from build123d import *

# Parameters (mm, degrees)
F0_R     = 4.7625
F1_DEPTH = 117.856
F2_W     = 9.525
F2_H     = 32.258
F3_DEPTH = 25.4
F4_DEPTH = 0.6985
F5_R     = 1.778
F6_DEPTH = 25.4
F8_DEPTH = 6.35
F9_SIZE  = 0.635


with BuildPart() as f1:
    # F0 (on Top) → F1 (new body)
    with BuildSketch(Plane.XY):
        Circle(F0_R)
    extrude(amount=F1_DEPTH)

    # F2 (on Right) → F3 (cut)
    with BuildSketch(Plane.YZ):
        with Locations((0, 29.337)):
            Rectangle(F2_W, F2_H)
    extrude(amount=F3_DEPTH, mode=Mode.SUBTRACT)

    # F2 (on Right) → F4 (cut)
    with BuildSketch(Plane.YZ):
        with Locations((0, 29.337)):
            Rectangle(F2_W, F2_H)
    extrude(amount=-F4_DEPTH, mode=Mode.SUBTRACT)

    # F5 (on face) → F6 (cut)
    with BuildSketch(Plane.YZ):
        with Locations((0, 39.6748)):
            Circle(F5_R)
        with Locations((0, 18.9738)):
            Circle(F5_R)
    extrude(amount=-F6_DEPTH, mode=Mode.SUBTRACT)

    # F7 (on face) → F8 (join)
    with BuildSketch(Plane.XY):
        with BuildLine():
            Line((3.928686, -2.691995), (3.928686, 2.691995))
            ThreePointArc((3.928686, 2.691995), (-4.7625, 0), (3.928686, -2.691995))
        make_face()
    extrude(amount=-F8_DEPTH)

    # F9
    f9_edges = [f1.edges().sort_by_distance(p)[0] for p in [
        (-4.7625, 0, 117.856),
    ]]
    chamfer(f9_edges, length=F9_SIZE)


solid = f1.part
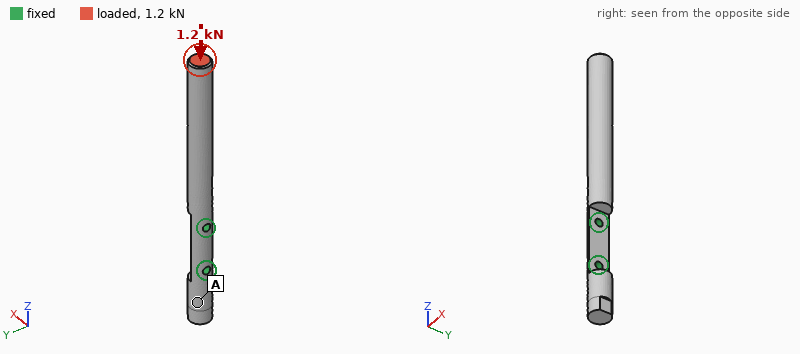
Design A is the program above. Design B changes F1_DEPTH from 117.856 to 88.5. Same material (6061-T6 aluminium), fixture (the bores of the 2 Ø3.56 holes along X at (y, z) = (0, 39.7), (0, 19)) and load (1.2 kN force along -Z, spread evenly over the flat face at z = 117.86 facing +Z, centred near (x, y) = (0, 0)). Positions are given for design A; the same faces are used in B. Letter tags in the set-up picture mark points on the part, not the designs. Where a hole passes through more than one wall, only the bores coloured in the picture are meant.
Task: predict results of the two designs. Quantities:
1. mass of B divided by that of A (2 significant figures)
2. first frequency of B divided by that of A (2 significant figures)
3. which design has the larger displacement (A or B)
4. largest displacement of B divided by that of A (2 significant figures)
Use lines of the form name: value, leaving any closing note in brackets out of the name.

mass of B divided by that of A: 0.72
first frequency of B divided by that of A: 2.2
which design has the larger displacement: A
largest displacement of B divided by that of A: 0.61
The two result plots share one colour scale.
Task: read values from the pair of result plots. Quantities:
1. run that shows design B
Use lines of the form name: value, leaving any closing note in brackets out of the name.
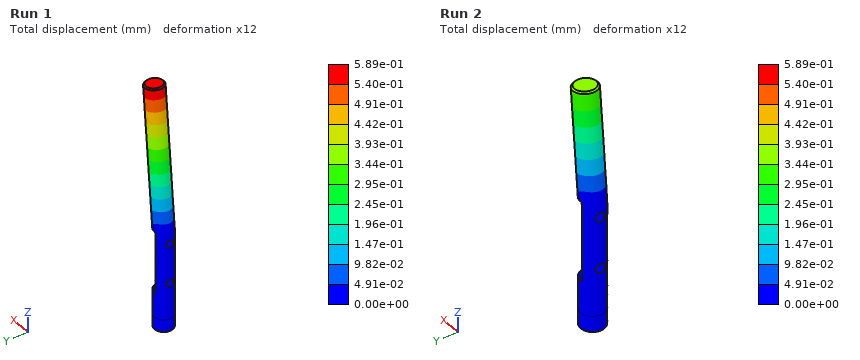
run that shows design B: Run 2
